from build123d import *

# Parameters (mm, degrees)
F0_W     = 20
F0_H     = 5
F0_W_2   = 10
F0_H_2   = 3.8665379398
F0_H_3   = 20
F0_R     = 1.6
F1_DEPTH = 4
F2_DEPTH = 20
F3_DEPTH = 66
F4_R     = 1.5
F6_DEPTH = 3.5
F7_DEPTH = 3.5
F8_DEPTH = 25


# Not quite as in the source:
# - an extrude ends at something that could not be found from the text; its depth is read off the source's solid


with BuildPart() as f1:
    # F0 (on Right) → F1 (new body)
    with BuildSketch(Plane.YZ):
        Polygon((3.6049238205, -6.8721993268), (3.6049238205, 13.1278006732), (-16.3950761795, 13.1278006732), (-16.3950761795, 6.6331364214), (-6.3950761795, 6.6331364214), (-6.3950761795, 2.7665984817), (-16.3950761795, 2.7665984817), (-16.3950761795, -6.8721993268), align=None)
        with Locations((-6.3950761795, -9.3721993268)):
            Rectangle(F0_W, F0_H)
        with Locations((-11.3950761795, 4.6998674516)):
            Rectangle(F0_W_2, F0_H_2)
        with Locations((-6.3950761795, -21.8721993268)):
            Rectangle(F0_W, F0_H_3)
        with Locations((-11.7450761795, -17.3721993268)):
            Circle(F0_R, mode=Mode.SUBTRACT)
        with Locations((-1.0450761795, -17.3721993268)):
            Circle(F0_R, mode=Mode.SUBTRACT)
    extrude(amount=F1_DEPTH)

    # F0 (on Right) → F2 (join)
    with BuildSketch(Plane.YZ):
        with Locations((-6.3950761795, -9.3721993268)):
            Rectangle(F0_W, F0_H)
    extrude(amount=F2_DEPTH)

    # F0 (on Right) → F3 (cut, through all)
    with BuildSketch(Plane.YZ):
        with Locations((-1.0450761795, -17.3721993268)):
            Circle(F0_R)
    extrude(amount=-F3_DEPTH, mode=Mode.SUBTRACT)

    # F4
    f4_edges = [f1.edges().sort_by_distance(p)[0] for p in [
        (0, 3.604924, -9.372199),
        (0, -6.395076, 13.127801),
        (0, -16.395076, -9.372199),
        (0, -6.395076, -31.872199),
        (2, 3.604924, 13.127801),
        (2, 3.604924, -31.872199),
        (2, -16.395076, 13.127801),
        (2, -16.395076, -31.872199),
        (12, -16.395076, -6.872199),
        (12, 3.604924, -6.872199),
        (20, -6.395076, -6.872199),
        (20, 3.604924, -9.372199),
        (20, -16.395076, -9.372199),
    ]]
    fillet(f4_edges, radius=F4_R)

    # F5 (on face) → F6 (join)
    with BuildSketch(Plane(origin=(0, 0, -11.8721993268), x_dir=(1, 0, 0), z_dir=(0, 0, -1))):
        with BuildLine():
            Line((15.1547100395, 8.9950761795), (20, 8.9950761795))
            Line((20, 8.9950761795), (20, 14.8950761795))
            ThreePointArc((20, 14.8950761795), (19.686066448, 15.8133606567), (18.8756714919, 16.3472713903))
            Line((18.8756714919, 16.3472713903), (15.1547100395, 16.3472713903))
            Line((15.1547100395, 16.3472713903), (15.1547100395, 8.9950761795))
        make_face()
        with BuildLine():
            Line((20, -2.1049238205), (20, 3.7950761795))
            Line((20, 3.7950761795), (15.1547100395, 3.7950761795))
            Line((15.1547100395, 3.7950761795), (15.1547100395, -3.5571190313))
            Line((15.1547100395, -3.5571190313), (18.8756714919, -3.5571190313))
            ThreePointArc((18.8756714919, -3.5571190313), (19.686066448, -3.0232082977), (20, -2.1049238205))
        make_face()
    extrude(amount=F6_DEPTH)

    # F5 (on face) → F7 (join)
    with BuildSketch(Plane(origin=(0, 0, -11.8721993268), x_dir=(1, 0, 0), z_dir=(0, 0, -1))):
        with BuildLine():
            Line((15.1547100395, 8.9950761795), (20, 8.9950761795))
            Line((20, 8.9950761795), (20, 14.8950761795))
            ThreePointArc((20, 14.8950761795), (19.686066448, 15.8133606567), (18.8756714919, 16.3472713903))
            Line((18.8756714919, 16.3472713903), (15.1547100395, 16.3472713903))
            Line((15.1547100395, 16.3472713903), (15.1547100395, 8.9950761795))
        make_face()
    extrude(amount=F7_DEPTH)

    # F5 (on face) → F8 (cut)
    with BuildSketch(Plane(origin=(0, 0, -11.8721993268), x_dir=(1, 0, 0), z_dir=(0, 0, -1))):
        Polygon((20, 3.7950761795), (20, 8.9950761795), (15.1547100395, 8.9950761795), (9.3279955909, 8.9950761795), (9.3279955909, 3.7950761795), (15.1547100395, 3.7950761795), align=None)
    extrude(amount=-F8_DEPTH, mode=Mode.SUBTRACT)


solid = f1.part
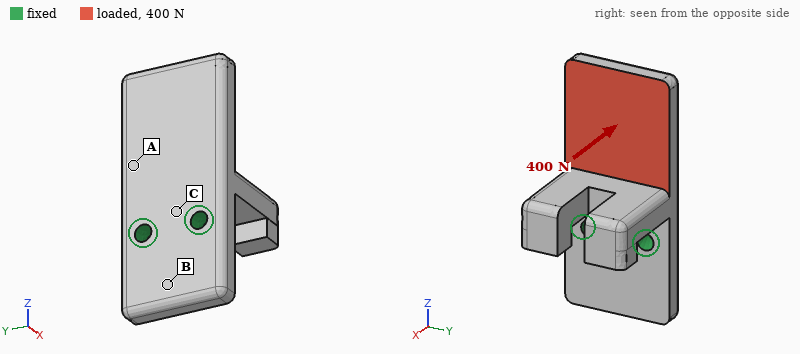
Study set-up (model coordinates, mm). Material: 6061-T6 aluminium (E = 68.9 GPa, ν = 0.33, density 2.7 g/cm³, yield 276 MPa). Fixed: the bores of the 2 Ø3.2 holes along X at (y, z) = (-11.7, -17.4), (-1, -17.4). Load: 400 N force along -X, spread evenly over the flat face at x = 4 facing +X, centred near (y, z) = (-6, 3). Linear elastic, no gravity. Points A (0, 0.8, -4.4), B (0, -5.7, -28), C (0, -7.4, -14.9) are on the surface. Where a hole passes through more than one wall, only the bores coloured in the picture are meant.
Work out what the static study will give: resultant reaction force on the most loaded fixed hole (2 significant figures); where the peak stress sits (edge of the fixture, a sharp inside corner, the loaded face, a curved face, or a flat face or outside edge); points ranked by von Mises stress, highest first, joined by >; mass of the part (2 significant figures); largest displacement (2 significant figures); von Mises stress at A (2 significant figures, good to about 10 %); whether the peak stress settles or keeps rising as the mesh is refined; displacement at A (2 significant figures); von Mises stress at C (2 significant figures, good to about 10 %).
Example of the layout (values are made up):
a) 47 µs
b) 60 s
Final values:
a) 200 N
b) edge of the fixture
c) C > A > B
d) 14 g
e) 0.24 mm
f) 56 MPa
g) keeps rising
h) 0.064 mm
i) 93 MPa
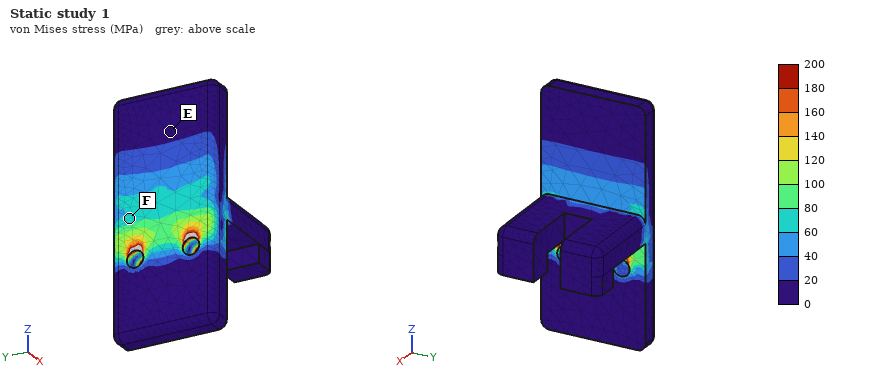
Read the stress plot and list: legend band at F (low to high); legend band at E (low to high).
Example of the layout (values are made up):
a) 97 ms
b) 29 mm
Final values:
a) 60 to 80 MPa
b) 0 to 20 MPa
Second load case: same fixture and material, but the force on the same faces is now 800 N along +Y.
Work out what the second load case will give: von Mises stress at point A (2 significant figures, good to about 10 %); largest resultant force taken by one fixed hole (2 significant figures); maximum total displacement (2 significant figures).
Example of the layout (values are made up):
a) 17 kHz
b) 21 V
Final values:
a) 22 MPa
b) 1.3 kN
c) 42 µm
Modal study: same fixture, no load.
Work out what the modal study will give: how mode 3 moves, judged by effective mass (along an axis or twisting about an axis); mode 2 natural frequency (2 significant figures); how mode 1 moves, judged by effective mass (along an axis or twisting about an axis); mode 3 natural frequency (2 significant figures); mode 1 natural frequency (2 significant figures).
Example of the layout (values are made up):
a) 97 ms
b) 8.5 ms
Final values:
a) along Z
b) 8900 Hz
c) along X
d) 9700 Hz
e) 3400 Hz
